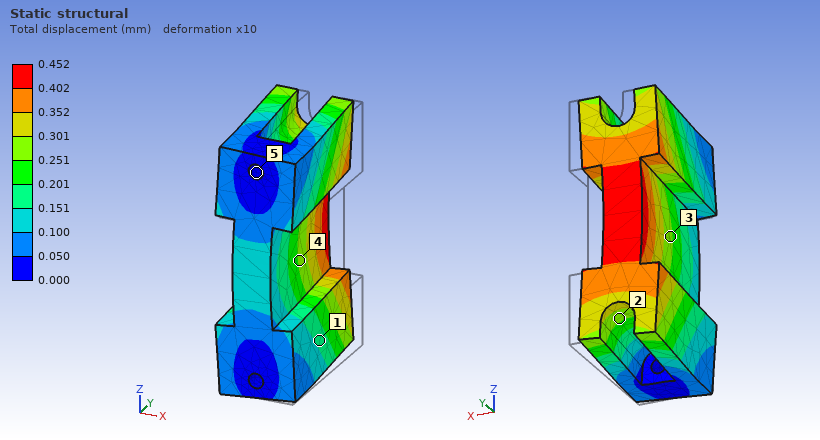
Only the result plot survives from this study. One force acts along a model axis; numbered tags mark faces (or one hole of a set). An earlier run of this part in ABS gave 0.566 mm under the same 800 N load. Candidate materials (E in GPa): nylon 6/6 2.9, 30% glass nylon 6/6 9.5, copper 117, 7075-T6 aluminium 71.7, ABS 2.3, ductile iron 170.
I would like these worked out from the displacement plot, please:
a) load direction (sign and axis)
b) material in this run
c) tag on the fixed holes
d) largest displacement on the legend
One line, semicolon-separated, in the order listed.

-X; nylon 6/6; 5; 0.452 mm
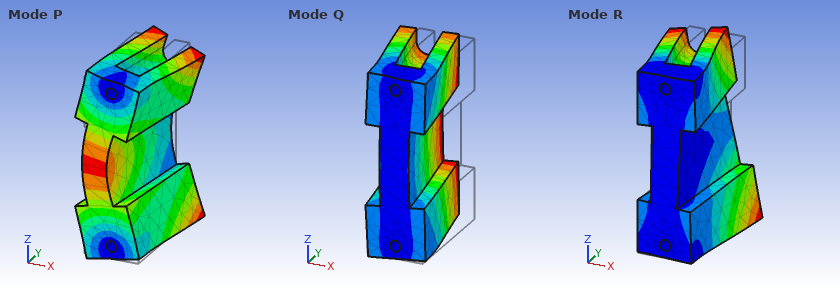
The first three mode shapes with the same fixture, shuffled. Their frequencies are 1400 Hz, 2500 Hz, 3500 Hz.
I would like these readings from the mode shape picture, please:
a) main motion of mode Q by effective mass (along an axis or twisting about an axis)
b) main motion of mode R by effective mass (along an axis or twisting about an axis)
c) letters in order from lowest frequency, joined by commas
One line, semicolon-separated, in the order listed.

along X; twisting about Y; Q, R, P
